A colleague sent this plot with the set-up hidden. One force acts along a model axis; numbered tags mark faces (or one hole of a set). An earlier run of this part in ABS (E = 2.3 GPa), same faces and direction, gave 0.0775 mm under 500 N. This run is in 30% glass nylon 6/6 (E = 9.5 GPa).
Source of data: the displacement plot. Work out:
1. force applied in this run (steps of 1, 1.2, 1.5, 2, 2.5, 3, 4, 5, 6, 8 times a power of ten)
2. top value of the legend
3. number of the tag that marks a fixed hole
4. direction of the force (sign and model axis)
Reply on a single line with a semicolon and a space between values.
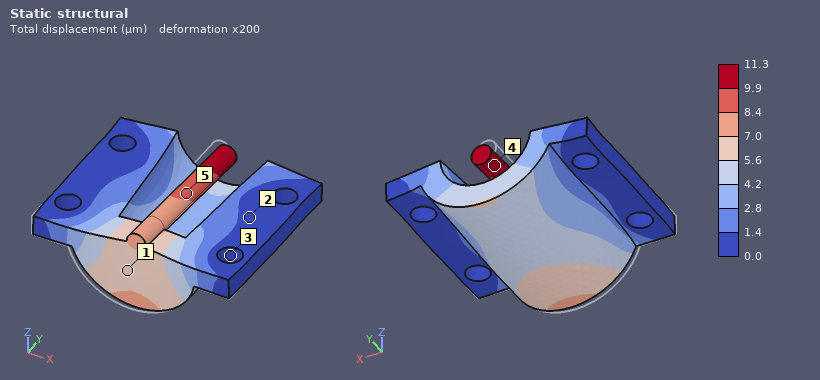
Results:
300 N; 11.3 µm; 3; +Y
